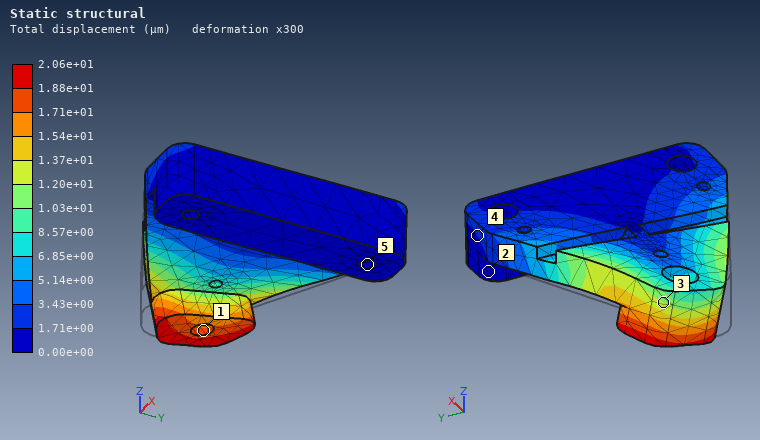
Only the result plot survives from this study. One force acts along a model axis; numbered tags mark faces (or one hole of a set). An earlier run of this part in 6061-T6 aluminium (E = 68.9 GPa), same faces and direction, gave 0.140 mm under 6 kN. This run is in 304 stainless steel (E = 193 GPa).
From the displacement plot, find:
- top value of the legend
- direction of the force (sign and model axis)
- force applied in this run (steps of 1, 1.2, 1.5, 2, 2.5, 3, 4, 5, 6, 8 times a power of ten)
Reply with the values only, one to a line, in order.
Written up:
2.06e+01 µm
+Y
2.5 kN
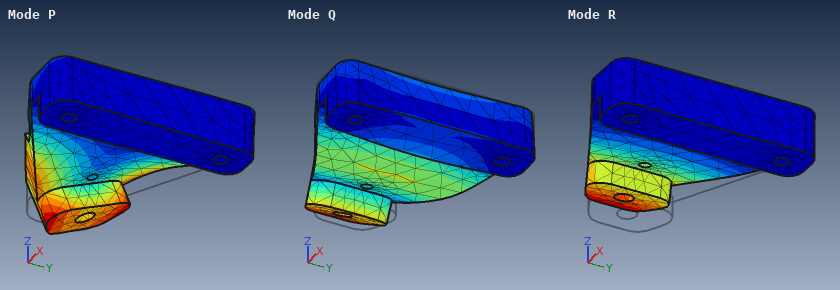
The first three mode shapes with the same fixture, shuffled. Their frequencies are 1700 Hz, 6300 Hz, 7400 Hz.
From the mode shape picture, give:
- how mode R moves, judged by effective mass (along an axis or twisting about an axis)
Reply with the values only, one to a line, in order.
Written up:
along Z
